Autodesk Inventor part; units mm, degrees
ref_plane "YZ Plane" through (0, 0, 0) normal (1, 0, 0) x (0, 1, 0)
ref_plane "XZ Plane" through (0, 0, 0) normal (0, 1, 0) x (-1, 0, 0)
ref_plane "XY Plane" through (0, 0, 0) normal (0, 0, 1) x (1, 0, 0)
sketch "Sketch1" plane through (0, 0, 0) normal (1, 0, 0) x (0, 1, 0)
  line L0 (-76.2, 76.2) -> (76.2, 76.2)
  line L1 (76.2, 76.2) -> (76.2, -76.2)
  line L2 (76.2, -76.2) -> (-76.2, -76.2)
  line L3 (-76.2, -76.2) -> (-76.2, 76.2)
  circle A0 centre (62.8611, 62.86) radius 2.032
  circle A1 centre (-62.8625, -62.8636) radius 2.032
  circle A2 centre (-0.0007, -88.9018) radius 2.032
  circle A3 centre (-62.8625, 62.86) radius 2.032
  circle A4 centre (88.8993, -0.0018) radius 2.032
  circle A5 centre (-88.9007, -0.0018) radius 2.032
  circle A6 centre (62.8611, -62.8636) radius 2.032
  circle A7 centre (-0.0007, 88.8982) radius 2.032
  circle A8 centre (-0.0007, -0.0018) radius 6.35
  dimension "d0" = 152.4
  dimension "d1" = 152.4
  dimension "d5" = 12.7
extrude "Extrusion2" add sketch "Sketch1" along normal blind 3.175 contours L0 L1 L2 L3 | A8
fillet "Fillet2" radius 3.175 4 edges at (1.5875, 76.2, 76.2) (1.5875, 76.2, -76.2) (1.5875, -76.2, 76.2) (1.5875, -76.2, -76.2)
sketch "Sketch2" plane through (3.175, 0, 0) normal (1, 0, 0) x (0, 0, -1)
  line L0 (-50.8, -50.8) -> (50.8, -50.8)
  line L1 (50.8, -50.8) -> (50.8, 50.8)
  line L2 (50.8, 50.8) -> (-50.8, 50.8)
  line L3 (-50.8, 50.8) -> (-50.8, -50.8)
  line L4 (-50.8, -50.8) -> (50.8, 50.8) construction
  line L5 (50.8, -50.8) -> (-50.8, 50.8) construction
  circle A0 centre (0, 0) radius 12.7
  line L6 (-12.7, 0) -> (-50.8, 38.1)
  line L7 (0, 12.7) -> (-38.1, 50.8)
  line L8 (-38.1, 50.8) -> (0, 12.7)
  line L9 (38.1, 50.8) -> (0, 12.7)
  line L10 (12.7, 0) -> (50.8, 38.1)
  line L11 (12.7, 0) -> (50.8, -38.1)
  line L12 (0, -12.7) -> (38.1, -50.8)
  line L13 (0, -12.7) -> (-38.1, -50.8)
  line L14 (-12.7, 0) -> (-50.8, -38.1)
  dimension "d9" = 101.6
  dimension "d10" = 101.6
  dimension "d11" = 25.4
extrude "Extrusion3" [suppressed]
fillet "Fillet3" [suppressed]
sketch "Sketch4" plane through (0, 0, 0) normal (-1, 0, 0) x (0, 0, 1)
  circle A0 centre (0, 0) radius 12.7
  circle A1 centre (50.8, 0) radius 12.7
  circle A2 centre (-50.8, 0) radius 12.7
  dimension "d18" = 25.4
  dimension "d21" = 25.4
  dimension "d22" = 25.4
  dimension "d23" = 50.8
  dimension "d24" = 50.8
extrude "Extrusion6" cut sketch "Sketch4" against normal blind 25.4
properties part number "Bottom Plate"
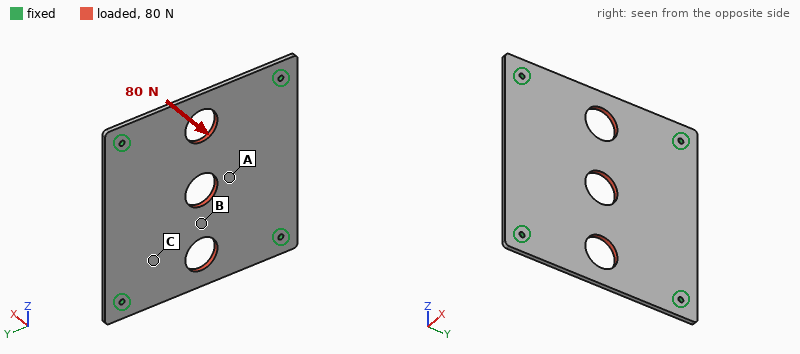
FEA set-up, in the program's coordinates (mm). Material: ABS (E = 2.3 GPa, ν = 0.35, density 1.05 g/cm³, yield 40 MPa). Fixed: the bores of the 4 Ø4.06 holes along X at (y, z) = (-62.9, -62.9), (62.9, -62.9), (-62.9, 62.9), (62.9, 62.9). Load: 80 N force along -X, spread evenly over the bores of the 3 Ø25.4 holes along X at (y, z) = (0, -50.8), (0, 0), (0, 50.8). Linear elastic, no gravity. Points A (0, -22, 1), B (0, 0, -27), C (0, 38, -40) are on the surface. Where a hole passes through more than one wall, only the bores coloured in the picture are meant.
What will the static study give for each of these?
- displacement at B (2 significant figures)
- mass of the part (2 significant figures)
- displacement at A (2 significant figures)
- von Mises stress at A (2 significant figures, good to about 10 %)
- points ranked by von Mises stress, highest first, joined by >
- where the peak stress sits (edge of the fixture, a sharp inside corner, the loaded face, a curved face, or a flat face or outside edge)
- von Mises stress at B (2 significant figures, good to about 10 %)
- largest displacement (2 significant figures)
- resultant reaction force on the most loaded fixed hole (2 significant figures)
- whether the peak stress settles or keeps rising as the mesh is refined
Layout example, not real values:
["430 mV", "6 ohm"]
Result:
["2.1 mm", "72 g", "1.9 mm", "3.1 MPa", "B > A > C", "edge of the fixture", "7.5 MPa", "2.4 mm", "20 N", "keeps rising"]
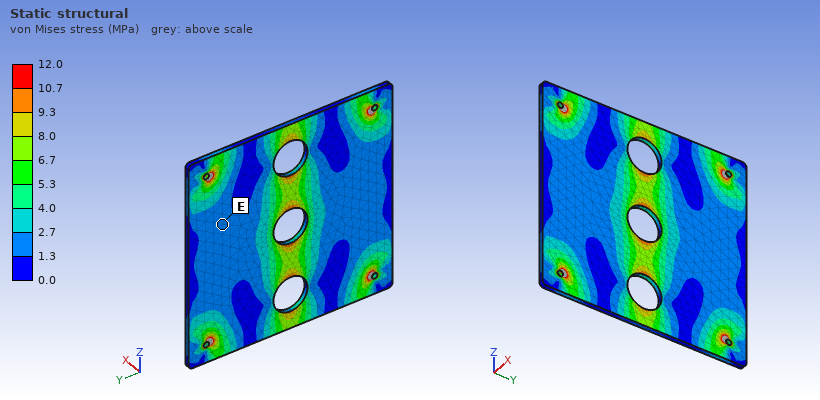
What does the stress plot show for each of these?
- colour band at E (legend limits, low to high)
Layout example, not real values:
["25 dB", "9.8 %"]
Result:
["1.3 to 2.7 MPa"]
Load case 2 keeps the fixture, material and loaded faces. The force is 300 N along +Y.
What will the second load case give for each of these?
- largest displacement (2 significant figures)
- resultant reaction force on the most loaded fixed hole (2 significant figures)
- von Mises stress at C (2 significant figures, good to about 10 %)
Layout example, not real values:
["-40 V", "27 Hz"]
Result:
["25 µm", "79 N", "0.47 MPa"]
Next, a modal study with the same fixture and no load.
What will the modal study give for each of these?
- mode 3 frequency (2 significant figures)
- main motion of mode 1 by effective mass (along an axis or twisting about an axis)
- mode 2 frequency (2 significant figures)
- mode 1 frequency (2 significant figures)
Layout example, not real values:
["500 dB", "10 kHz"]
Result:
["330 Hz", "along X", "320 Hz", "190 Hz"]
